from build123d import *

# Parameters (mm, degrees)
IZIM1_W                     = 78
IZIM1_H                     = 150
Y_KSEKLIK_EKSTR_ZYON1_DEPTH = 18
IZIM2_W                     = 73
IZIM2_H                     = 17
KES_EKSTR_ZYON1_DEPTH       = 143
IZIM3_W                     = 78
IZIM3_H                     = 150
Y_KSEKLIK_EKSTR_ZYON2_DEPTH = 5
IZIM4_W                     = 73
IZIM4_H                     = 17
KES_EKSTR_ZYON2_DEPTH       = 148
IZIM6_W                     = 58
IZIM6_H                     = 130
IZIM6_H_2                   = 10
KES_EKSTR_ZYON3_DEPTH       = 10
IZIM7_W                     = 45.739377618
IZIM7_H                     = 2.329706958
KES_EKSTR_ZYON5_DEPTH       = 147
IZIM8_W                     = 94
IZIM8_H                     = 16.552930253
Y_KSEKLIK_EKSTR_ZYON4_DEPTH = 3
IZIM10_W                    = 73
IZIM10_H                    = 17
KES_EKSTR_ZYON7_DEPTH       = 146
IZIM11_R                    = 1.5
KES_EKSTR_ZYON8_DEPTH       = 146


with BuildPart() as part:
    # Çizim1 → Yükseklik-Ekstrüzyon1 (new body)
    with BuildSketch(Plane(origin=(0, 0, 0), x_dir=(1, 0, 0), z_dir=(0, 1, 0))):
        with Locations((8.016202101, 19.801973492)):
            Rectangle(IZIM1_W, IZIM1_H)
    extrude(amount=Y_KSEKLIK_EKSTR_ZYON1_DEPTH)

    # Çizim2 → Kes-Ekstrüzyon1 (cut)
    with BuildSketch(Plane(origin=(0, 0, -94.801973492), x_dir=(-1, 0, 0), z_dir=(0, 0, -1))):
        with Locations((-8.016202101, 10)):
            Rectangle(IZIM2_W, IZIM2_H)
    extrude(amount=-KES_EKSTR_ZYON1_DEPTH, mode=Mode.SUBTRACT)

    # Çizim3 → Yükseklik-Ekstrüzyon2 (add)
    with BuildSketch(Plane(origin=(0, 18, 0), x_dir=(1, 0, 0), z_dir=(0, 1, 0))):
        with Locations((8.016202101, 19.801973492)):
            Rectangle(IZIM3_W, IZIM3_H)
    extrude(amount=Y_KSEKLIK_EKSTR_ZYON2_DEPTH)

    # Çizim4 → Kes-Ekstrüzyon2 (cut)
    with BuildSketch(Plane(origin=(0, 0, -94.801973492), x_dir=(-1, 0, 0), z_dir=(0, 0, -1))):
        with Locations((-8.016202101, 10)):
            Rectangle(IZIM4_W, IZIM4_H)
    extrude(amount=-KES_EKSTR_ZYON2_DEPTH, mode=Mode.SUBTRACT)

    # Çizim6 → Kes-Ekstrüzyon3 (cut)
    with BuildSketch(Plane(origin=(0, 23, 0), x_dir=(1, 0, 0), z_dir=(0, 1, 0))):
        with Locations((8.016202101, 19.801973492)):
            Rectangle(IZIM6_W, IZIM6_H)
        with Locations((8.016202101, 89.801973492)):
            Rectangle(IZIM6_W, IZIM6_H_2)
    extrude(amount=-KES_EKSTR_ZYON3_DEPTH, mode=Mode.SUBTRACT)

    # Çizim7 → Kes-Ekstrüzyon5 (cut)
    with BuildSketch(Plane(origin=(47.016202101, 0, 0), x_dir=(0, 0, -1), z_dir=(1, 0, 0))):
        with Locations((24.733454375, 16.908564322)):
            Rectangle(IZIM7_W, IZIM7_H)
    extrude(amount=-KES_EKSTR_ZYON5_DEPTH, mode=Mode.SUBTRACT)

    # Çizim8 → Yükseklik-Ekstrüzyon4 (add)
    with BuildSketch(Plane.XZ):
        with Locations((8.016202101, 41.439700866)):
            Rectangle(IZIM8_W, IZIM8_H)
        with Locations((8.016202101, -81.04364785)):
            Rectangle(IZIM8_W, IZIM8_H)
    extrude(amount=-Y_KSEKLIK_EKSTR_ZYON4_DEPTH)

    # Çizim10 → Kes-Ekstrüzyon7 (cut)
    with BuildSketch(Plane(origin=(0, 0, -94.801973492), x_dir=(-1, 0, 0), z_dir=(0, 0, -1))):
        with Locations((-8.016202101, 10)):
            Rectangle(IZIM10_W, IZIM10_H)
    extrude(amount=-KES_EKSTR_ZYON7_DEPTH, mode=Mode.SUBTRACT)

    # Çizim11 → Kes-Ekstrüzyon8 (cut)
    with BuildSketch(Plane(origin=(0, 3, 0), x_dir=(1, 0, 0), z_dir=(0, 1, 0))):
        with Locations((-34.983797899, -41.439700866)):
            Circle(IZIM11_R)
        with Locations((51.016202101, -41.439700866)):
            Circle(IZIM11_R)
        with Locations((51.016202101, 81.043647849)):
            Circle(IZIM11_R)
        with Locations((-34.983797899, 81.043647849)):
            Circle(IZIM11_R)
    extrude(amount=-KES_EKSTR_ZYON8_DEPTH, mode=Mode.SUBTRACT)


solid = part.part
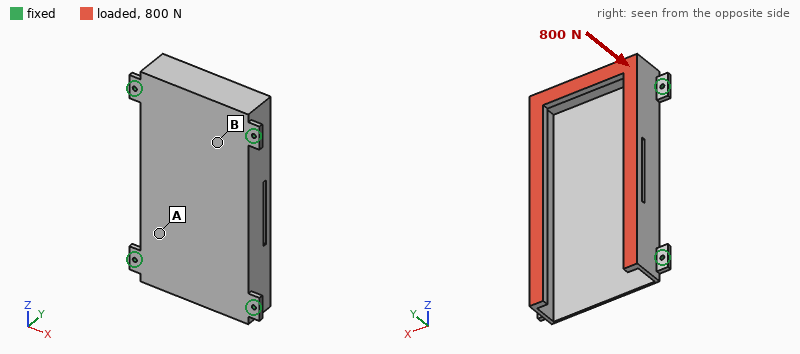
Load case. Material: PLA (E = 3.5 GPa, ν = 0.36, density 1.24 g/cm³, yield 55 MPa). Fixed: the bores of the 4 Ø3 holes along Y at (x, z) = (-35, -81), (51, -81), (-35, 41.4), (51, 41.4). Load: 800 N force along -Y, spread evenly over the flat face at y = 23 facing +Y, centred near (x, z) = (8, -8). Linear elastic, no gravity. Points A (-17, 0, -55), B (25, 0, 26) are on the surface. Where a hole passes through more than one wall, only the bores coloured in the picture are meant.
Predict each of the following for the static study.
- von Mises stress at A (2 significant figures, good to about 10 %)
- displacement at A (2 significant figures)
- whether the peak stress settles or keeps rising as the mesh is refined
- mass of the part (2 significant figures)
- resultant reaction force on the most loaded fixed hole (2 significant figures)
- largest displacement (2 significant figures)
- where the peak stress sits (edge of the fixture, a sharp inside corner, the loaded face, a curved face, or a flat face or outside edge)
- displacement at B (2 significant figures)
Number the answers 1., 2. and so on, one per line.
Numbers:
1. 4.1 MPa
2. 0.66 mm
3. keeps rising
4. 62 g
5. 250 N
6. 1.5 mm
7. edge of the fixture
8. 0.33 mm
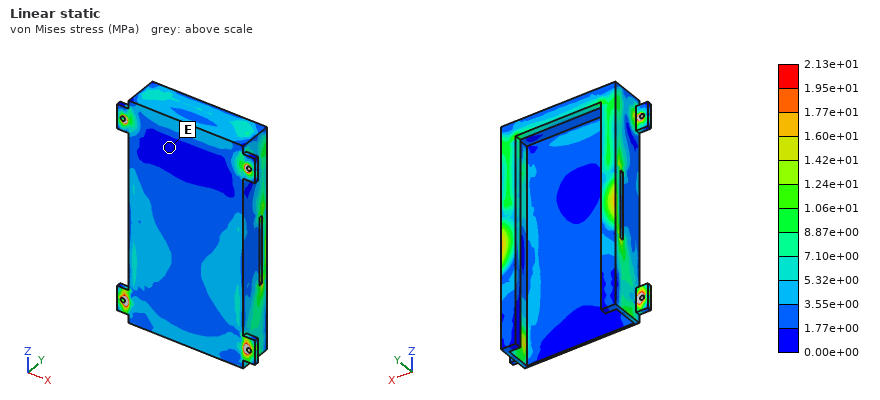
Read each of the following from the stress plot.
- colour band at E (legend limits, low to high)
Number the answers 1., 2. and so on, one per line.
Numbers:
1. 0.00e+00 to 1.77e+00 MPa
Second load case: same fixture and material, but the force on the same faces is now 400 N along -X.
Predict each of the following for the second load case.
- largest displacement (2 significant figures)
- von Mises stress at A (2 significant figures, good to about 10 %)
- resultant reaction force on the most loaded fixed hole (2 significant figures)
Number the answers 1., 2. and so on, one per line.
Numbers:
1. 2.1 mm
2. 10 MPa
3. 140 N
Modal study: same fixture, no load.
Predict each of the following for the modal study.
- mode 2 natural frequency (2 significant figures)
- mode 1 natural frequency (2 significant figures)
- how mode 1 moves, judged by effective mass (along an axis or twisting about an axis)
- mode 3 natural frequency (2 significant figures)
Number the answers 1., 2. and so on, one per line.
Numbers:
1. 520 Hz
2. 360 Hz
3. along Y
4. 530 Hz
